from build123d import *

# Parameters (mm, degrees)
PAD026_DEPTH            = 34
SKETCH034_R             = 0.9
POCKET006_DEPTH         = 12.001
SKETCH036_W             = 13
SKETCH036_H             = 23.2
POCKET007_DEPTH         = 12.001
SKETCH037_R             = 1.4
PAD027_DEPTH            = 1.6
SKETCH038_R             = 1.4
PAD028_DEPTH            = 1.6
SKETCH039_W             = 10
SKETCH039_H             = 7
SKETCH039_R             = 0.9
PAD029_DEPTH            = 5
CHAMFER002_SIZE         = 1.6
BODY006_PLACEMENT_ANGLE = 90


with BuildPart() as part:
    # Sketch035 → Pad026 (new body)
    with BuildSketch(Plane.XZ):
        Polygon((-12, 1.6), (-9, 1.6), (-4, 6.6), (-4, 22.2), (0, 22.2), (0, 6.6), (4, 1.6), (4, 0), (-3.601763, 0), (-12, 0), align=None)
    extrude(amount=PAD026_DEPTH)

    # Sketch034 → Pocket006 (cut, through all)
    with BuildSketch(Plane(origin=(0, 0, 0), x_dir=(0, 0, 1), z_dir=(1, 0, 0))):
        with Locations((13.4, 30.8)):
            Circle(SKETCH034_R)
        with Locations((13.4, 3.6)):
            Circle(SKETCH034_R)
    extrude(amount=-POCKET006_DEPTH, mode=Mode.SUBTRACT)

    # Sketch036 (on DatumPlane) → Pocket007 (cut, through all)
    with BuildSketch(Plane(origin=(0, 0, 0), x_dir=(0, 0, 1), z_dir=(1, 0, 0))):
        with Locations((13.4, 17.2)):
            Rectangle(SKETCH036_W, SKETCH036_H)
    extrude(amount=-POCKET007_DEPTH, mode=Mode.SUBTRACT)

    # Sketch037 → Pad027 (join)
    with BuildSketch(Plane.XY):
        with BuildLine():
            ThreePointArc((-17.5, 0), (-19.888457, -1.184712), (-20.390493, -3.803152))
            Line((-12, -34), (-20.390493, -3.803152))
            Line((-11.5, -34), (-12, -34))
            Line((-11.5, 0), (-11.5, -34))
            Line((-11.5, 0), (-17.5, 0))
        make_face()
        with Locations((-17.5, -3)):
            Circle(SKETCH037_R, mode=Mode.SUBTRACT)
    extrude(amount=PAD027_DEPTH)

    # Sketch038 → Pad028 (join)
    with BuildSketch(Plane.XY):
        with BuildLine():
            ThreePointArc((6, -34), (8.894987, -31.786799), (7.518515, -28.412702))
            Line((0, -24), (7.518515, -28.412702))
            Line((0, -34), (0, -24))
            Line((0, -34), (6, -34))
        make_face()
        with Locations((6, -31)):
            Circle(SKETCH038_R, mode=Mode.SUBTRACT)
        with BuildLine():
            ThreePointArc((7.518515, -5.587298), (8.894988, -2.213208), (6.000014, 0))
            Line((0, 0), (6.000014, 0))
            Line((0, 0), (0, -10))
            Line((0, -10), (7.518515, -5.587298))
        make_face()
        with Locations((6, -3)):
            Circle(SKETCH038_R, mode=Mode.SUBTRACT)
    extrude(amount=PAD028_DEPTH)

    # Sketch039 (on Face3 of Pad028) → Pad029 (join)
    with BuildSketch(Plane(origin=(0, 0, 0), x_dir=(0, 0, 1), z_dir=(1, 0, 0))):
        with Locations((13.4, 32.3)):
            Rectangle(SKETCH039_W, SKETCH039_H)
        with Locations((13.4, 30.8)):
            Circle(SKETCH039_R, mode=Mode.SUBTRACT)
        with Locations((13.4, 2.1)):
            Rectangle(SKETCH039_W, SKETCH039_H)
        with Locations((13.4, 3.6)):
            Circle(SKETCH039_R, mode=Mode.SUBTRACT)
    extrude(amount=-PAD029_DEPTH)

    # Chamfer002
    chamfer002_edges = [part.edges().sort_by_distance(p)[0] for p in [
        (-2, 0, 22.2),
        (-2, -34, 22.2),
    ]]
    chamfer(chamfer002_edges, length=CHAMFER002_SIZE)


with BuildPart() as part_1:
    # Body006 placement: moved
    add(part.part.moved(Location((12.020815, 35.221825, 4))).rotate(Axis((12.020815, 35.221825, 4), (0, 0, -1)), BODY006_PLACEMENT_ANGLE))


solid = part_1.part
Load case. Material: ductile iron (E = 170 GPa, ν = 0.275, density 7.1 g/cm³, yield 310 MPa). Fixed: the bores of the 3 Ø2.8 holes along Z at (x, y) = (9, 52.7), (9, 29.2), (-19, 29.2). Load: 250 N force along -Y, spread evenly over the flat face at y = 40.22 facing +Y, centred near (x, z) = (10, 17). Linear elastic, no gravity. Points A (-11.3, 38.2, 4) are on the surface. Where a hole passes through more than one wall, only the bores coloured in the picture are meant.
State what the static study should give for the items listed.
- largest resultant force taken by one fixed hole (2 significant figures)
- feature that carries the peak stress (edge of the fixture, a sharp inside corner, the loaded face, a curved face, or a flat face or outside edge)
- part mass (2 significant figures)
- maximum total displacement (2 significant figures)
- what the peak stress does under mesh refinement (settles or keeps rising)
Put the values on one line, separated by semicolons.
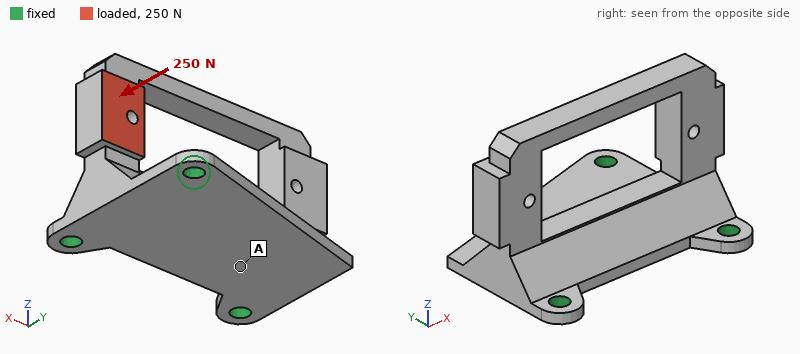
200 N; edge of the fixture; 27 g; 45 µm; keeps rising
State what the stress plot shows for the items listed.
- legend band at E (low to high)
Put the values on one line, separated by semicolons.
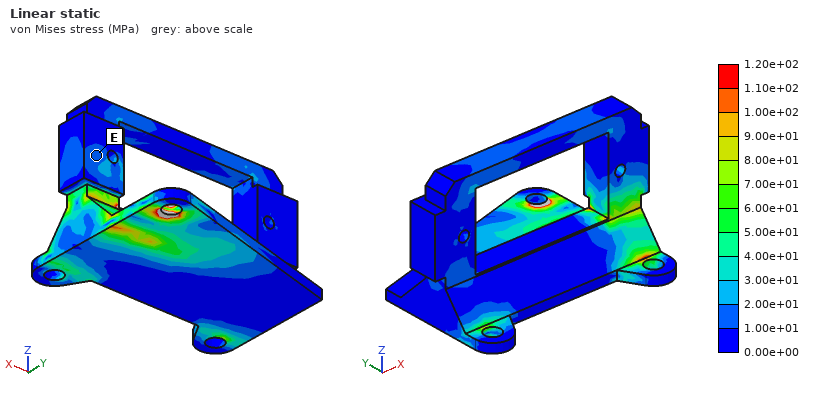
1.00e+01 to 2.00e+01 MPa
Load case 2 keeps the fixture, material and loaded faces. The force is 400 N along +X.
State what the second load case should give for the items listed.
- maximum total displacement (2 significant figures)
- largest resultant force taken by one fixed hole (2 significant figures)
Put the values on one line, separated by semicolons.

21 µm; 260 N
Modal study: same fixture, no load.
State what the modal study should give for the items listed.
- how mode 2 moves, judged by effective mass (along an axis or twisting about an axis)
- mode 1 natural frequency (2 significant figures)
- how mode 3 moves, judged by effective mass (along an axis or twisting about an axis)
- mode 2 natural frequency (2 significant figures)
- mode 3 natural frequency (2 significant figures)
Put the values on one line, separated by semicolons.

along X; 3800 Hz; along X; 7300 Hz; 9500 Hz
